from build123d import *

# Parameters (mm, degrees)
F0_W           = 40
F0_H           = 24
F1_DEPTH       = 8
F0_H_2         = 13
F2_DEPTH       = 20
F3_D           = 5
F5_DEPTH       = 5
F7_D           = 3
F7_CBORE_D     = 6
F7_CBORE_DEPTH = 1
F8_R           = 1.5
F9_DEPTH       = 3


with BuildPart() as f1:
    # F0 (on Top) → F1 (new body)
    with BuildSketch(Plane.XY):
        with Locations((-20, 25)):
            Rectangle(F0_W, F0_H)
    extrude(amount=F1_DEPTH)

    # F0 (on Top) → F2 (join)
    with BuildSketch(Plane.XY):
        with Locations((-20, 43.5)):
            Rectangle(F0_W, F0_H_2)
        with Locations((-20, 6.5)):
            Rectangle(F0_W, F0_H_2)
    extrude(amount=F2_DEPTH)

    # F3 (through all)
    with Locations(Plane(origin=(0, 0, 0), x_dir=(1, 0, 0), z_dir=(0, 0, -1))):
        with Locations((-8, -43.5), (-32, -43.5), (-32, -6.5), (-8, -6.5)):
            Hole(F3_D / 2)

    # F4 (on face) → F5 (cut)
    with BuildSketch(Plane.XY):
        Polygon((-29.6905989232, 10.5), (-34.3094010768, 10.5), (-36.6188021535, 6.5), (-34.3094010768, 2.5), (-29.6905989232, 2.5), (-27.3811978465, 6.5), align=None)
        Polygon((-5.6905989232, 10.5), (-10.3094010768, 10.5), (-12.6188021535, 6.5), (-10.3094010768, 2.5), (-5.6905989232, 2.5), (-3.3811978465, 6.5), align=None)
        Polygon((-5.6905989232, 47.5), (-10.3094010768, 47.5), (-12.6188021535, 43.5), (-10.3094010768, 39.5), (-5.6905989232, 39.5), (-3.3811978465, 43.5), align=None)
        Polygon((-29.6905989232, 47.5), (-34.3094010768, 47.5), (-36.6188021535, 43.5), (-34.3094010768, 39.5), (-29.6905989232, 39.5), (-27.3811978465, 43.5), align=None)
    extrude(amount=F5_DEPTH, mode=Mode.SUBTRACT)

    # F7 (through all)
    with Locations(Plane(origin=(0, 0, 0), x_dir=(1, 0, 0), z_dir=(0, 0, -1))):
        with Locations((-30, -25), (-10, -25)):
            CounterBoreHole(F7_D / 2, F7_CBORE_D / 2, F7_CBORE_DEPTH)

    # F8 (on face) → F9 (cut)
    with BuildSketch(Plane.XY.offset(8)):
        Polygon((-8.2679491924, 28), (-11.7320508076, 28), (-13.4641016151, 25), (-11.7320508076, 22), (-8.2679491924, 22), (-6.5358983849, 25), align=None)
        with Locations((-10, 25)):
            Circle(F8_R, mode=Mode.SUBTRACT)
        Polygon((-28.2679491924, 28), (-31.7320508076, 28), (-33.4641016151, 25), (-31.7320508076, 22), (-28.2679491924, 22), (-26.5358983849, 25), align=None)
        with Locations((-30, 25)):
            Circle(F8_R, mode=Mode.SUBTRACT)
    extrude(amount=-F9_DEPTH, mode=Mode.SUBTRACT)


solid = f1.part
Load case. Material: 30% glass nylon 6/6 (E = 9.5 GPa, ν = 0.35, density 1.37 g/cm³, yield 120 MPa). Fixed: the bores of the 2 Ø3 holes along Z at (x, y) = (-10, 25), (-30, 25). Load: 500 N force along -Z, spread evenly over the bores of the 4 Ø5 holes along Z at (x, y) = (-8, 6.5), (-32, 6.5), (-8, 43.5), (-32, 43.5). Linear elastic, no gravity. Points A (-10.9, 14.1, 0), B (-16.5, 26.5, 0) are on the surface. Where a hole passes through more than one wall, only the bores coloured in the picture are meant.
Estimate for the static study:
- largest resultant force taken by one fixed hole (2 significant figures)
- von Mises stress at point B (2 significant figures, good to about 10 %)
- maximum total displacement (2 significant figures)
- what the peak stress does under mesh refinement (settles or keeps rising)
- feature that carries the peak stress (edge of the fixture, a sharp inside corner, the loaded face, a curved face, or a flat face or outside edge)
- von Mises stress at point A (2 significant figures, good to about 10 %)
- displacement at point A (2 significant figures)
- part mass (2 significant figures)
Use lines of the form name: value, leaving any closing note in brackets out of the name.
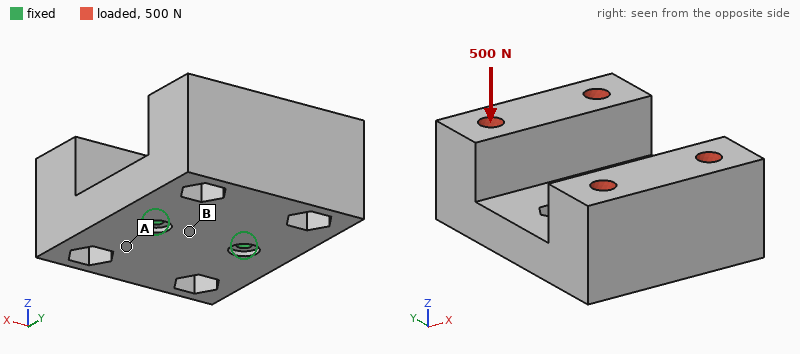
largest resultant force taken by one fixed hole: 250 N
von Mises stress at point B: 10 MPa
maximum total displacement: 78 µm
what the peak stress does under mesh refinement: keeps rising
feature that carries the peak stress: edge of the fixture
von Mises stress at point A: 3.2 MPa
displacement at point A: 23 µm
part mass: 35 g
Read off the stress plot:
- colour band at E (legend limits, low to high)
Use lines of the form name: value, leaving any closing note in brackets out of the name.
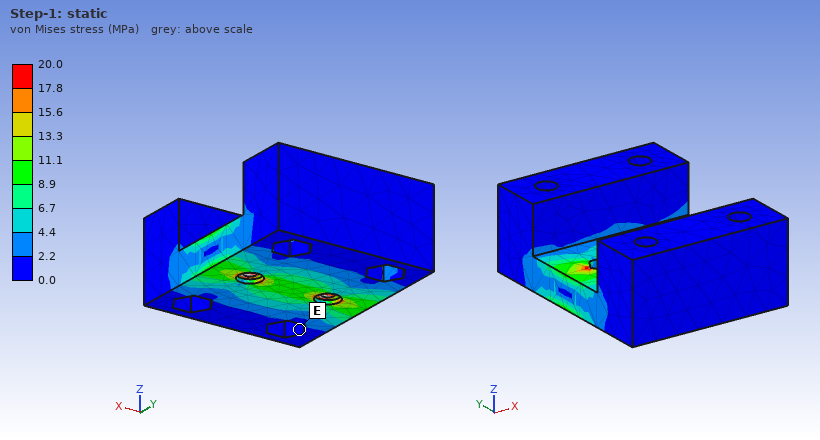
colour band at E: 0.0 to 2.2 MPa
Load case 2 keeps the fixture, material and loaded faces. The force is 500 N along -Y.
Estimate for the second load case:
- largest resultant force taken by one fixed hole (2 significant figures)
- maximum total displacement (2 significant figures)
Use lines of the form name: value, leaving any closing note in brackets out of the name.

largest resultant force taken by one fixed hole: 250 N
maximum total displacement: 0.22 mm
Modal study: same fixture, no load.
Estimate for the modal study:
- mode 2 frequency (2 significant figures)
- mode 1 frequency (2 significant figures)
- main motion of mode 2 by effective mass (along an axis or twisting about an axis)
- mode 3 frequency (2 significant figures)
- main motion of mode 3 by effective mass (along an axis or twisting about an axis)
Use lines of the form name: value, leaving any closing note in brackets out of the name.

mode 2 frequency: 2800 Hz
mode 1 frequency: 1300 Hz
main motion of mode 2 by effective mass: along Z
mode 3 frequency: 4200 Hz
main motion of mode 3 by effective mass: along X
